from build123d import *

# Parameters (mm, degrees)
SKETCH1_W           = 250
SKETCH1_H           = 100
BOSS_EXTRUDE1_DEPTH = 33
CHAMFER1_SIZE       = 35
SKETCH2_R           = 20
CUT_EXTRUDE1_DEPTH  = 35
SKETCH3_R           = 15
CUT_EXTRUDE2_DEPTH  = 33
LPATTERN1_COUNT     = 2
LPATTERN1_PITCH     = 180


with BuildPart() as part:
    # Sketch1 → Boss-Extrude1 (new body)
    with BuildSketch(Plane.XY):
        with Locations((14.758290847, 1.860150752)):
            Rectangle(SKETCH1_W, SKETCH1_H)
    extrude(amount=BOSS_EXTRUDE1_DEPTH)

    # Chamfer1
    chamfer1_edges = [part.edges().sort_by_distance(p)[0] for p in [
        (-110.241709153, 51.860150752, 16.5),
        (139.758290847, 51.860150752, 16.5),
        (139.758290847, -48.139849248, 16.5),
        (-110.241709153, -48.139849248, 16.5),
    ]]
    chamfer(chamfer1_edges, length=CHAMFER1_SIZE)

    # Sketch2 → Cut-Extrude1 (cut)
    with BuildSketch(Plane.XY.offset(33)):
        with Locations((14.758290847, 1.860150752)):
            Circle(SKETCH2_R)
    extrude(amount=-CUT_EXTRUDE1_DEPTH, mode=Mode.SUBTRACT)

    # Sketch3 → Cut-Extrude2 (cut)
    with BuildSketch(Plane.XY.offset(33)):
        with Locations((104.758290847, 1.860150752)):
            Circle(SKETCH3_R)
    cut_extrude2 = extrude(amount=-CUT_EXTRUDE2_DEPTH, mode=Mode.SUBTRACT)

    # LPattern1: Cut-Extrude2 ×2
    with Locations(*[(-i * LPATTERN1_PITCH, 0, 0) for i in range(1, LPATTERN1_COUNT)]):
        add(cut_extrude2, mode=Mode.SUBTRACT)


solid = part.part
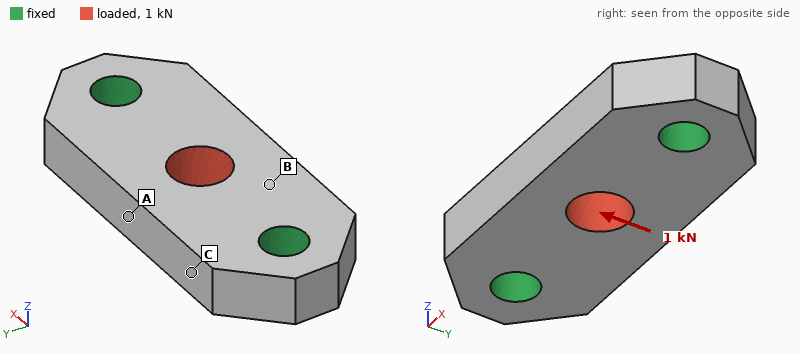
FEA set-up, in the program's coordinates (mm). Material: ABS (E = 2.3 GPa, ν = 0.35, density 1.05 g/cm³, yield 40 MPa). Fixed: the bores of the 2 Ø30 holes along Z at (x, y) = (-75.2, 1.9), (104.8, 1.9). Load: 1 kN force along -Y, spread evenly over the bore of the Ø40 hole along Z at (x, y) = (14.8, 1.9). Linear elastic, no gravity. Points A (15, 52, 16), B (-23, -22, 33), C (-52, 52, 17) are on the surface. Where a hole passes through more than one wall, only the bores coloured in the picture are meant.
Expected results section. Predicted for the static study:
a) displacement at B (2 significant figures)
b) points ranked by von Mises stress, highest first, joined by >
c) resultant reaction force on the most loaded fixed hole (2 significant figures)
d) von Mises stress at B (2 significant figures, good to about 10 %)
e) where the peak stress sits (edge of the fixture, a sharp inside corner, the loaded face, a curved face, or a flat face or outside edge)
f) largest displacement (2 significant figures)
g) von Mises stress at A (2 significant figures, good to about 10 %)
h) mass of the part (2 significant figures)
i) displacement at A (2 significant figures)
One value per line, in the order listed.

16 µm
A > B > C
500 N
0.33 MPa
edge of the fixture
25 µm
0.62 MPa
690 g
22 µm
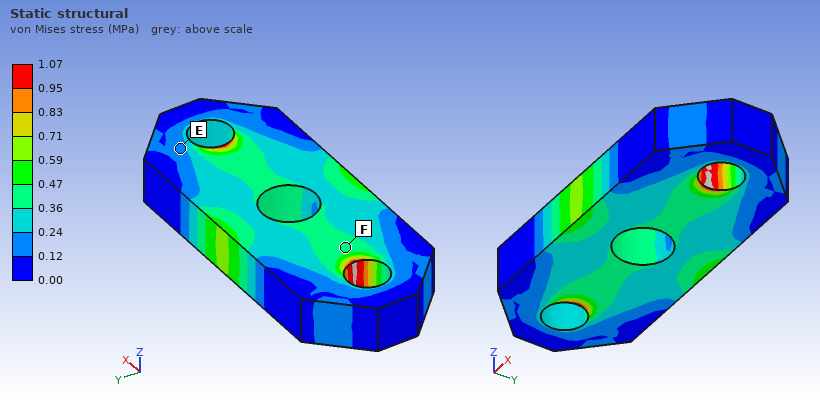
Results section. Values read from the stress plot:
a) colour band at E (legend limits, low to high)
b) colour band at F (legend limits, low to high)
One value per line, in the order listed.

0.12 to 0.24 MPa
0.36 to 0.47 MPa
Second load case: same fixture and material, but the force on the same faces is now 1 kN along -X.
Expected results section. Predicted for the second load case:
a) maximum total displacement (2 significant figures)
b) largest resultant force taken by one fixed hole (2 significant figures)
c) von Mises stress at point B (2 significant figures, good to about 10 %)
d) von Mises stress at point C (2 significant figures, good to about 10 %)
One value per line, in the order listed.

7.8 µm
500 N
0.19 MPa
0.033 MPa
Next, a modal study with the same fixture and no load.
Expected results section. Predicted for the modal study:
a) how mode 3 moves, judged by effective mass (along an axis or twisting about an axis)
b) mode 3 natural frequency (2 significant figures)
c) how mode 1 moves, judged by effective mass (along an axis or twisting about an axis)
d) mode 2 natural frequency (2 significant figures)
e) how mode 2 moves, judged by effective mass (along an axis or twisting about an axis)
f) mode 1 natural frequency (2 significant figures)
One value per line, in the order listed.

along Y
2100 Hz
along Z
1500 Hz
twisting about X
1400 Hz
